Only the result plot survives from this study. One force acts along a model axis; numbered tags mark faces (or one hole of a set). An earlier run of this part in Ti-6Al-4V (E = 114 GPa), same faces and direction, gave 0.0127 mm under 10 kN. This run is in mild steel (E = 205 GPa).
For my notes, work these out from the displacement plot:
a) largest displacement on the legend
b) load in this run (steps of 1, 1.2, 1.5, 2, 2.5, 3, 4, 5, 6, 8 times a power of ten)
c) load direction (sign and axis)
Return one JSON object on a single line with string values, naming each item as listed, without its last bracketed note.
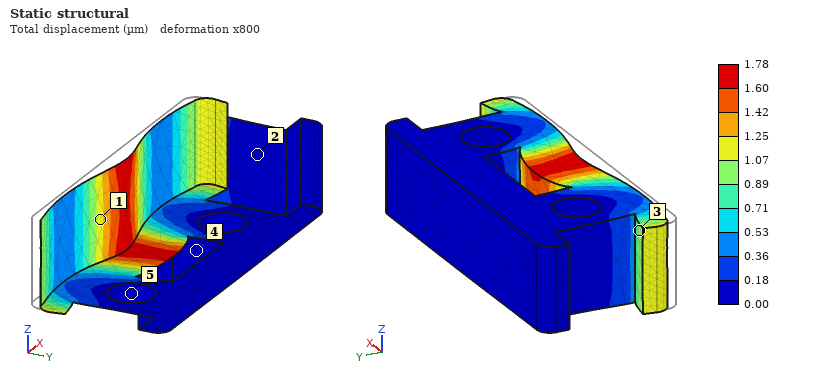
{"largest displacement on the legend": "1.78 µm", "load in this run": "2.5 kN", "load direction": "+Y"}
